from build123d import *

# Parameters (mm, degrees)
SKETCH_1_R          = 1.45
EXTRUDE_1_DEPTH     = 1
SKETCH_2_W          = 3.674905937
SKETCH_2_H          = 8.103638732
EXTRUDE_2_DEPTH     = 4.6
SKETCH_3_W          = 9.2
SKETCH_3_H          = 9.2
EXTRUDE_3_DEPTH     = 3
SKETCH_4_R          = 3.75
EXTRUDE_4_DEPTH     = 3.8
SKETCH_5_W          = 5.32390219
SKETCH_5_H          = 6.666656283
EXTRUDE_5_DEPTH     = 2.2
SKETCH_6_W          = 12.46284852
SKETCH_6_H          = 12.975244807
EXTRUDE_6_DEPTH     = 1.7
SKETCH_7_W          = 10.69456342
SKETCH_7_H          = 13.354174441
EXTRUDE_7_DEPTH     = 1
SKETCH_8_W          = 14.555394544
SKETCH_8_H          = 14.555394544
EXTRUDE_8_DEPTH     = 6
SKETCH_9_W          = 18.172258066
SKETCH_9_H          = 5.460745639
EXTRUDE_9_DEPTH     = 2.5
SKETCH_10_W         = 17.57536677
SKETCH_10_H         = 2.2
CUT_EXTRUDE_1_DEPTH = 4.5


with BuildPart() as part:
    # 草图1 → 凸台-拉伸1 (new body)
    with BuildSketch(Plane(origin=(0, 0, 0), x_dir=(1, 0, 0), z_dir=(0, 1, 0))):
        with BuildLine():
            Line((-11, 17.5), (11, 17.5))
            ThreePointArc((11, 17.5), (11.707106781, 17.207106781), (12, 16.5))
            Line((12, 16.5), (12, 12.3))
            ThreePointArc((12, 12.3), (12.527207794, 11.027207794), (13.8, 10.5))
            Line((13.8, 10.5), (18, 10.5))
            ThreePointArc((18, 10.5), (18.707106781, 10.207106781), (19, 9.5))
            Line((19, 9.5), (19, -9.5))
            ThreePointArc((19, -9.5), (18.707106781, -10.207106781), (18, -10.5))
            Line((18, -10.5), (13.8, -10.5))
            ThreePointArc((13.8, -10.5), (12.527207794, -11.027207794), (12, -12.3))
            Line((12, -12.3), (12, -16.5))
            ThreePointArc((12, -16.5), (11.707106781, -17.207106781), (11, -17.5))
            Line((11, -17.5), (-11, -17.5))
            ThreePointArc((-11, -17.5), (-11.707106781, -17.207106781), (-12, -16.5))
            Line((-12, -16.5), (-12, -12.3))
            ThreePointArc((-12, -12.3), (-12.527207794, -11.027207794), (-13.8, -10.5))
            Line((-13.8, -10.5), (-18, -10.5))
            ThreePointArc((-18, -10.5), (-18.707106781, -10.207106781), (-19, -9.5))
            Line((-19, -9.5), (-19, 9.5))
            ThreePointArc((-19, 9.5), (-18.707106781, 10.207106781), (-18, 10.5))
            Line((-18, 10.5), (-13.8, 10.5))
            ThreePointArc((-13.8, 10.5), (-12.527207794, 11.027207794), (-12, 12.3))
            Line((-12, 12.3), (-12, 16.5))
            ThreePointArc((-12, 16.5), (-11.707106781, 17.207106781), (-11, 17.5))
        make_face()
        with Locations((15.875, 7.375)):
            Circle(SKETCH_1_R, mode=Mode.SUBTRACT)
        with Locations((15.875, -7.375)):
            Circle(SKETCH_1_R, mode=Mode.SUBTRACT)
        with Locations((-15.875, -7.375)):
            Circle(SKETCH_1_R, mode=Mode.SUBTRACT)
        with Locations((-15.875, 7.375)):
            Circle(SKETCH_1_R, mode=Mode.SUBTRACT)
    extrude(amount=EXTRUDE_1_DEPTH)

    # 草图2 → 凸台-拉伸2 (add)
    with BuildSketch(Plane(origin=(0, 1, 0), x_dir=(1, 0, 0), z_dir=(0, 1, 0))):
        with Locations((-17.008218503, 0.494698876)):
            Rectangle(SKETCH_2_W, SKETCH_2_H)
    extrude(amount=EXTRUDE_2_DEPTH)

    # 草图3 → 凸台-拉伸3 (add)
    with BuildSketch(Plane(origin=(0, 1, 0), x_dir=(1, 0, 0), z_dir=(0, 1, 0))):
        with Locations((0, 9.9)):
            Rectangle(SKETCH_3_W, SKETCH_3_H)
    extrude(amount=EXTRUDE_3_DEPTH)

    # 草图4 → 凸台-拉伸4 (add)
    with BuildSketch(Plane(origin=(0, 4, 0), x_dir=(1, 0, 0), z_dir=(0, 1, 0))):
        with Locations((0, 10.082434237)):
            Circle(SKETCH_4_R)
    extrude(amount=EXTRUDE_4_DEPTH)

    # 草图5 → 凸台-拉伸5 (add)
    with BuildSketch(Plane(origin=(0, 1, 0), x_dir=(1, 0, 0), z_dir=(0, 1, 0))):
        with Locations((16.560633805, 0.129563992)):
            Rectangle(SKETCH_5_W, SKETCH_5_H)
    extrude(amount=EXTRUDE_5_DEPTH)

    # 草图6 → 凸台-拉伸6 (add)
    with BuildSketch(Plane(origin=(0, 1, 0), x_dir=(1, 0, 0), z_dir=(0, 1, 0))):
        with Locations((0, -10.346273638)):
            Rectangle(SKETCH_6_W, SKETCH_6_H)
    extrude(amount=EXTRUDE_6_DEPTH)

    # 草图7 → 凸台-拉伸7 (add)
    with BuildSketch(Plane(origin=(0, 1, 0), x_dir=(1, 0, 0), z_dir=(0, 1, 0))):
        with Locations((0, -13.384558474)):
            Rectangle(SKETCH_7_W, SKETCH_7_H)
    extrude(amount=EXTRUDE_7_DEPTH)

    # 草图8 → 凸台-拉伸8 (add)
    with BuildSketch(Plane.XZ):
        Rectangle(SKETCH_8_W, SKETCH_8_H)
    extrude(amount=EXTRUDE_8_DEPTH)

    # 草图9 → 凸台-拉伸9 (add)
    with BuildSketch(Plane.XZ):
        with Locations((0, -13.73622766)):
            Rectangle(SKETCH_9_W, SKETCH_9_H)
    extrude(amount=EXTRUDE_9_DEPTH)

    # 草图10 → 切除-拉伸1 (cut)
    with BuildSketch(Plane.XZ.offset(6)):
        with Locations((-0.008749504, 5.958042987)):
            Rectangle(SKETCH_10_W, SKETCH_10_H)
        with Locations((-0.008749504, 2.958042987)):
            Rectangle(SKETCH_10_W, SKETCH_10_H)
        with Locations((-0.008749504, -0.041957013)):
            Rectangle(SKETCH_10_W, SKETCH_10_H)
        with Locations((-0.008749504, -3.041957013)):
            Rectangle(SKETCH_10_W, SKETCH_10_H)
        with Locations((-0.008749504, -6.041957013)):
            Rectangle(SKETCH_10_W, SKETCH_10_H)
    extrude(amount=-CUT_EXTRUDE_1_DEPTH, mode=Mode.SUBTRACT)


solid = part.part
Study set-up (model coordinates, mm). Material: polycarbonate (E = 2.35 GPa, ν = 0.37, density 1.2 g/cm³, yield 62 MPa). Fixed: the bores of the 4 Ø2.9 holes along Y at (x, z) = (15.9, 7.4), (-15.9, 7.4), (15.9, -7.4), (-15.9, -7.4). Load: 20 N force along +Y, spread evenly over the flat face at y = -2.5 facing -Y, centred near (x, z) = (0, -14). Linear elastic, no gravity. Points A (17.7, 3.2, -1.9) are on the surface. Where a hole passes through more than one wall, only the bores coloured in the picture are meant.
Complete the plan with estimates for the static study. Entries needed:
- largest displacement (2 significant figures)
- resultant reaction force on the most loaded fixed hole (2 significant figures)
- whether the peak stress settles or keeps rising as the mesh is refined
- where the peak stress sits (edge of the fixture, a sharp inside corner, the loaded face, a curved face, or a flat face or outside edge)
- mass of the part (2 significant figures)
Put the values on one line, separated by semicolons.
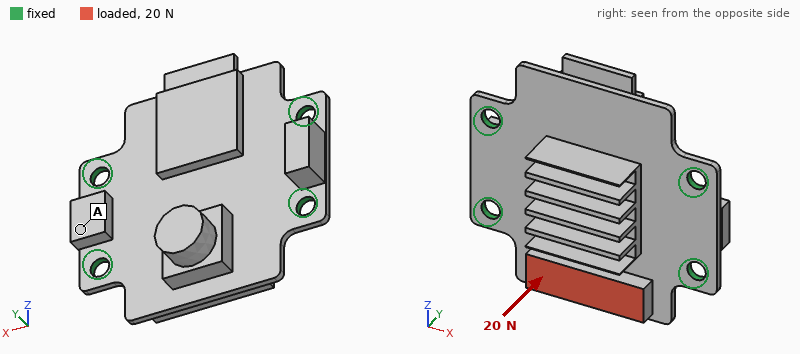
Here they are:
0.57 mm; 15 N; keeps rising; edge of the fixture; 3.4 g
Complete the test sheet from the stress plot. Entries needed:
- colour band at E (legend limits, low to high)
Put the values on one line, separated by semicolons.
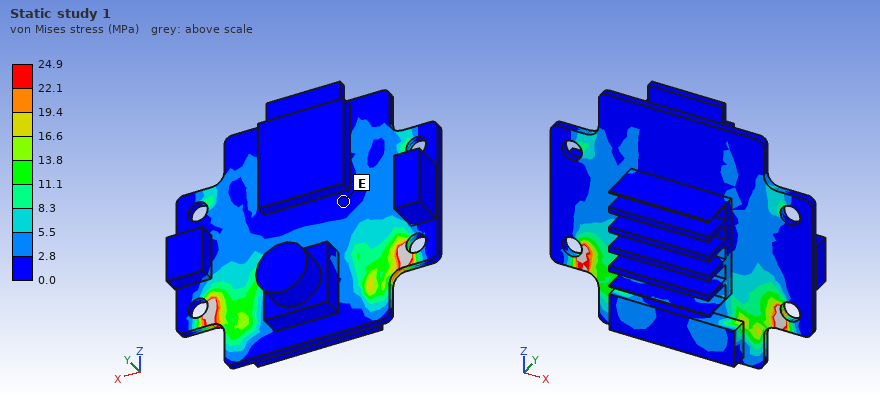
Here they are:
0.0 to 2.8 MPa
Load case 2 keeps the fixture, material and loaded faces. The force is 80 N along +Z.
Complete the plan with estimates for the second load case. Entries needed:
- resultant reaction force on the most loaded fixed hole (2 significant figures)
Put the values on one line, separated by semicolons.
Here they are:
22 N
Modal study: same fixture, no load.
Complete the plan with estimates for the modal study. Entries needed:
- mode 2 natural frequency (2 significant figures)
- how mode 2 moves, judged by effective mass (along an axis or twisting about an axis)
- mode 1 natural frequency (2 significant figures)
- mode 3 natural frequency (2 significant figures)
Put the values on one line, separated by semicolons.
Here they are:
1300 Hz; along Y; 1000 Hz; 2600 Hz
